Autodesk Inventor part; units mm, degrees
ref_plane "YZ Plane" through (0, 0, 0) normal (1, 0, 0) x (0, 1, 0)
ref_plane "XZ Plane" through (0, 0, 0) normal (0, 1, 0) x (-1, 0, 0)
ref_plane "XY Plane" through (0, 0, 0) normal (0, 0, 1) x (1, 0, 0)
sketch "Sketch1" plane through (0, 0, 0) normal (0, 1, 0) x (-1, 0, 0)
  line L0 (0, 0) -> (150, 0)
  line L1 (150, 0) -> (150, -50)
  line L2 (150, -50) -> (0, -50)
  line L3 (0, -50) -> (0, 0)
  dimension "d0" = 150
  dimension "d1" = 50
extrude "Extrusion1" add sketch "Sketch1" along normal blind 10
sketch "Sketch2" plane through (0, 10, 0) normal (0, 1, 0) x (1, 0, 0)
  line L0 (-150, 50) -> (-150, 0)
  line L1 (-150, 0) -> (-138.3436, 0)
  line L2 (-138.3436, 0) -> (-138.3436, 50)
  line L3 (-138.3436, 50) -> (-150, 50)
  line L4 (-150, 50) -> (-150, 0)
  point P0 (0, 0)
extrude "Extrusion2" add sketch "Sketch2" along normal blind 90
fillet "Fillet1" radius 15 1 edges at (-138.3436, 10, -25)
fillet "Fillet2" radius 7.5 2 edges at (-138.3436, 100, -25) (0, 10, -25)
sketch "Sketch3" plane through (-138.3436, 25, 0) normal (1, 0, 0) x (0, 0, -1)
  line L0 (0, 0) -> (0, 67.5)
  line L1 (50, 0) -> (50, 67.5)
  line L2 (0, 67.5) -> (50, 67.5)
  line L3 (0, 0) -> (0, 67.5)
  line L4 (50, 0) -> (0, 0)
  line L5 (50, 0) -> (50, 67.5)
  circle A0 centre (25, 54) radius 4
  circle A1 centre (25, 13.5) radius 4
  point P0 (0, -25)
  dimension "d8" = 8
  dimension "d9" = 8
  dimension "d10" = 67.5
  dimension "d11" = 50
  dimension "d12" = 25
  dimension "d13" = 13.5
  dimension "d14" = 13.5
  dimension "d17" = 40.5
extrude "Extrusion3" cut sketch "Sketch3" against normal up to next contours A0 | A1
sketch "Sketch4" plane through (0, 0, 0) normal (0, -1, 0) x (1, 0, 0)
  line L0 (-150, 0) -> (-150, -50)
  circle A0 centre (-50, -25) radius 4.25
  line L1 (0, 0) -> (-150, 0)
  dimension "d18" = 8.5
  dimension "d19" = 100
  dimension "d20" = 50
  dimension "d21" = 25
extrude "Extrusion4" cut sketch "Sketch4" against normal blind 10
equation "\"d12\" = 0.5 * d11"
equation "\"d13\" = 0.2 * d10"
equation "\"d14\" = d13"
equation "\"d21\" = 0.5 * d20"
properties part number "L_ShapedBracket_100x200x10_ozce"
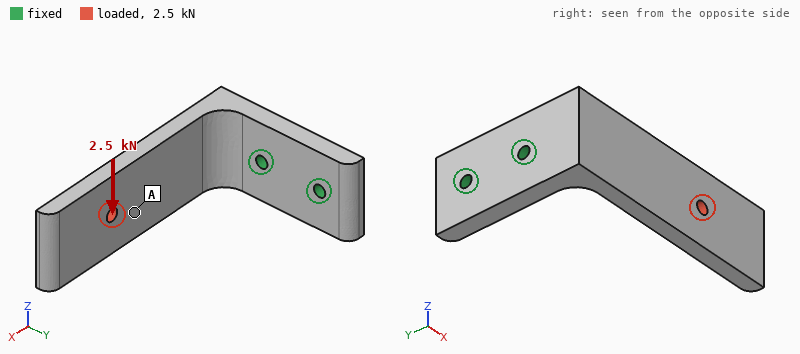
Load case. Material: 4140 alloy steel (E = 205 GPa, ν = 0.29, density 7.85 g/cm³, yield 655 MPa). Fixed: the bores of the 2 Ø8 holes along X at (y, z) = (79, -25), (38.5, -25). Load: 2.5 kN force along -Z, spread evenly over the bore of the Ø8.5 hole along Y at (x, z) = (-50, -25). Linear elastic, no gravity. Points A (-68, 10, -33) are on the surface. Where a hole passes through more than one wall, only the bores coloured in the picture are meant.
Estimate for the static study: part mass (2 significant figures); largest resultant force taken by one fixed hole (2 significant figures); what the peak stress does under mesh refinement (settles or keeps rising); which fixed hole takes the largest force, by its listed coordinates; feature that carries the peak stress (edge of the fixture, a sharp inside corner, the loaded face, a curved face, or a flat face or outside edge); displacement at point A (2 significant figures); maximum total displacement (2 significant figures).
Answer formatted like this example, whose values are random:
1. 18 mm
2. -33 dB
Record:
1. 1000 g
2. 4.1 kN
3. keeps rising
4. (38.5, -25)
5. edge of the fixture
6. 0.26 mm
7. 0.51 mm
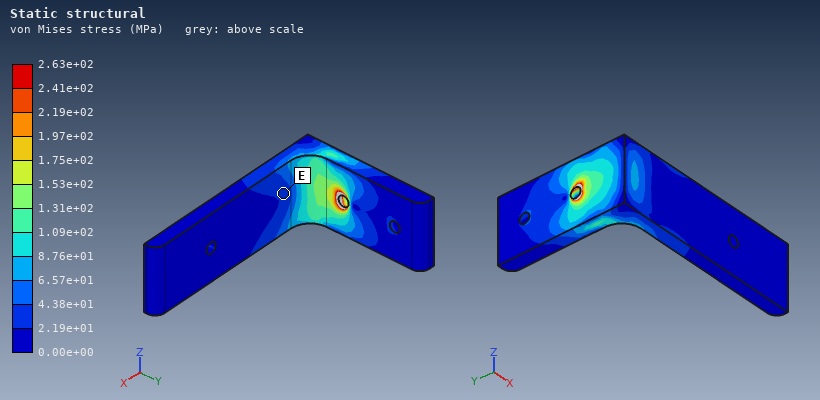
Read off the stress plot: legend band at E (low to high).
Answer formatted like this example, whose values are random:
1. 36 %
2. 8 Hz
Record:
1. 2.19e+01 to 4.38e+01 MPa
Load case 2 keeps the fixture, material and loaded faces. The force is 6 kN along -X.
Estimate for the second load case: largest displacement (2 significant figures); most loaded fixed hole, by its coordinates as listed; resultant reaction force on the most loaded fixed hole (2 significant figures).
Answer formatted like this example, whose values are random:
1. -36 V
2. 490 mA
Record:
1. 0.38 mm
2. (38.5, -25)
3. 7.7 kN
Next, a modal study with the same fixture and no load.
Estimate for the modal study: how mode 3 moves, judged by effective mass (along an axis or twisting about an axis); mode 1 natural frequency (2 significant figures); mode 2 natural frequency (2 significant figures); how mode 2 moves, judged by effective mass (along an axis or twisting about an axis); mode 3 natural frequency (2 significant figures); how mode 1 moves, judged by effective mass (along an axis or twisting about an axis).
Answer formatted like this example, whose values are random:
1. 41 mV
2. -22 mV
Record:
1. along X
2. 370 Hz
3. 660 Hz
4. along Z
5. 1800 Hz
6. along Y
